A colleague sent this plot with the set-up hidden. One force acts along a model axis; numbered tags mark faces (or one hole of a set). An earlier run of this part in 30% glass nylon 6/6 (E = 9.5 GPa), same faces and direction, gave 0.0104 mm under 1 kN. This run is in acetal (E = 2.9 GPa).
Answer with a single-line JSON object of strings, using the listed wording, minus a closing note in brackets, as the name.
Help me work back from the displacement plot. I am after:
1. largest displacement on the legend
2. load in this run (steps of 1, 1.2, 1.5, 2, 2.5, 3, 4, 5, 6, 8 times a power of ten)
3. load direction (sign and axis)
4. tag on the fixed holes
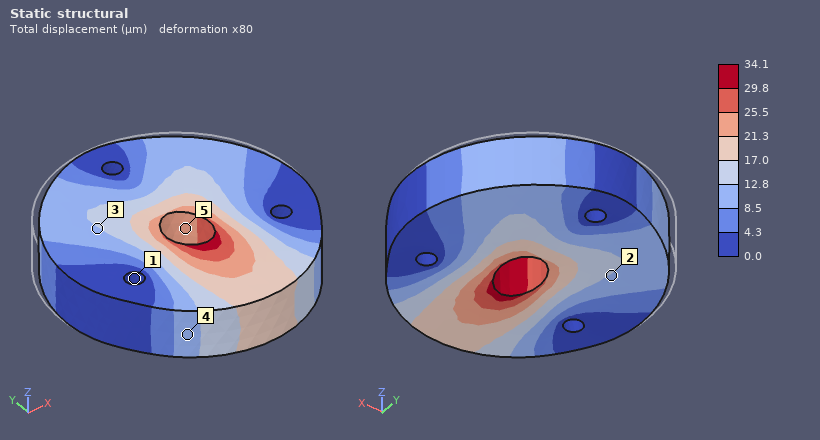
{"largest displacement on the legend": "34.1 µm", "load in this run": "1 kN", "load direction": "-Y", "tag on the fixed holes": "1"}
